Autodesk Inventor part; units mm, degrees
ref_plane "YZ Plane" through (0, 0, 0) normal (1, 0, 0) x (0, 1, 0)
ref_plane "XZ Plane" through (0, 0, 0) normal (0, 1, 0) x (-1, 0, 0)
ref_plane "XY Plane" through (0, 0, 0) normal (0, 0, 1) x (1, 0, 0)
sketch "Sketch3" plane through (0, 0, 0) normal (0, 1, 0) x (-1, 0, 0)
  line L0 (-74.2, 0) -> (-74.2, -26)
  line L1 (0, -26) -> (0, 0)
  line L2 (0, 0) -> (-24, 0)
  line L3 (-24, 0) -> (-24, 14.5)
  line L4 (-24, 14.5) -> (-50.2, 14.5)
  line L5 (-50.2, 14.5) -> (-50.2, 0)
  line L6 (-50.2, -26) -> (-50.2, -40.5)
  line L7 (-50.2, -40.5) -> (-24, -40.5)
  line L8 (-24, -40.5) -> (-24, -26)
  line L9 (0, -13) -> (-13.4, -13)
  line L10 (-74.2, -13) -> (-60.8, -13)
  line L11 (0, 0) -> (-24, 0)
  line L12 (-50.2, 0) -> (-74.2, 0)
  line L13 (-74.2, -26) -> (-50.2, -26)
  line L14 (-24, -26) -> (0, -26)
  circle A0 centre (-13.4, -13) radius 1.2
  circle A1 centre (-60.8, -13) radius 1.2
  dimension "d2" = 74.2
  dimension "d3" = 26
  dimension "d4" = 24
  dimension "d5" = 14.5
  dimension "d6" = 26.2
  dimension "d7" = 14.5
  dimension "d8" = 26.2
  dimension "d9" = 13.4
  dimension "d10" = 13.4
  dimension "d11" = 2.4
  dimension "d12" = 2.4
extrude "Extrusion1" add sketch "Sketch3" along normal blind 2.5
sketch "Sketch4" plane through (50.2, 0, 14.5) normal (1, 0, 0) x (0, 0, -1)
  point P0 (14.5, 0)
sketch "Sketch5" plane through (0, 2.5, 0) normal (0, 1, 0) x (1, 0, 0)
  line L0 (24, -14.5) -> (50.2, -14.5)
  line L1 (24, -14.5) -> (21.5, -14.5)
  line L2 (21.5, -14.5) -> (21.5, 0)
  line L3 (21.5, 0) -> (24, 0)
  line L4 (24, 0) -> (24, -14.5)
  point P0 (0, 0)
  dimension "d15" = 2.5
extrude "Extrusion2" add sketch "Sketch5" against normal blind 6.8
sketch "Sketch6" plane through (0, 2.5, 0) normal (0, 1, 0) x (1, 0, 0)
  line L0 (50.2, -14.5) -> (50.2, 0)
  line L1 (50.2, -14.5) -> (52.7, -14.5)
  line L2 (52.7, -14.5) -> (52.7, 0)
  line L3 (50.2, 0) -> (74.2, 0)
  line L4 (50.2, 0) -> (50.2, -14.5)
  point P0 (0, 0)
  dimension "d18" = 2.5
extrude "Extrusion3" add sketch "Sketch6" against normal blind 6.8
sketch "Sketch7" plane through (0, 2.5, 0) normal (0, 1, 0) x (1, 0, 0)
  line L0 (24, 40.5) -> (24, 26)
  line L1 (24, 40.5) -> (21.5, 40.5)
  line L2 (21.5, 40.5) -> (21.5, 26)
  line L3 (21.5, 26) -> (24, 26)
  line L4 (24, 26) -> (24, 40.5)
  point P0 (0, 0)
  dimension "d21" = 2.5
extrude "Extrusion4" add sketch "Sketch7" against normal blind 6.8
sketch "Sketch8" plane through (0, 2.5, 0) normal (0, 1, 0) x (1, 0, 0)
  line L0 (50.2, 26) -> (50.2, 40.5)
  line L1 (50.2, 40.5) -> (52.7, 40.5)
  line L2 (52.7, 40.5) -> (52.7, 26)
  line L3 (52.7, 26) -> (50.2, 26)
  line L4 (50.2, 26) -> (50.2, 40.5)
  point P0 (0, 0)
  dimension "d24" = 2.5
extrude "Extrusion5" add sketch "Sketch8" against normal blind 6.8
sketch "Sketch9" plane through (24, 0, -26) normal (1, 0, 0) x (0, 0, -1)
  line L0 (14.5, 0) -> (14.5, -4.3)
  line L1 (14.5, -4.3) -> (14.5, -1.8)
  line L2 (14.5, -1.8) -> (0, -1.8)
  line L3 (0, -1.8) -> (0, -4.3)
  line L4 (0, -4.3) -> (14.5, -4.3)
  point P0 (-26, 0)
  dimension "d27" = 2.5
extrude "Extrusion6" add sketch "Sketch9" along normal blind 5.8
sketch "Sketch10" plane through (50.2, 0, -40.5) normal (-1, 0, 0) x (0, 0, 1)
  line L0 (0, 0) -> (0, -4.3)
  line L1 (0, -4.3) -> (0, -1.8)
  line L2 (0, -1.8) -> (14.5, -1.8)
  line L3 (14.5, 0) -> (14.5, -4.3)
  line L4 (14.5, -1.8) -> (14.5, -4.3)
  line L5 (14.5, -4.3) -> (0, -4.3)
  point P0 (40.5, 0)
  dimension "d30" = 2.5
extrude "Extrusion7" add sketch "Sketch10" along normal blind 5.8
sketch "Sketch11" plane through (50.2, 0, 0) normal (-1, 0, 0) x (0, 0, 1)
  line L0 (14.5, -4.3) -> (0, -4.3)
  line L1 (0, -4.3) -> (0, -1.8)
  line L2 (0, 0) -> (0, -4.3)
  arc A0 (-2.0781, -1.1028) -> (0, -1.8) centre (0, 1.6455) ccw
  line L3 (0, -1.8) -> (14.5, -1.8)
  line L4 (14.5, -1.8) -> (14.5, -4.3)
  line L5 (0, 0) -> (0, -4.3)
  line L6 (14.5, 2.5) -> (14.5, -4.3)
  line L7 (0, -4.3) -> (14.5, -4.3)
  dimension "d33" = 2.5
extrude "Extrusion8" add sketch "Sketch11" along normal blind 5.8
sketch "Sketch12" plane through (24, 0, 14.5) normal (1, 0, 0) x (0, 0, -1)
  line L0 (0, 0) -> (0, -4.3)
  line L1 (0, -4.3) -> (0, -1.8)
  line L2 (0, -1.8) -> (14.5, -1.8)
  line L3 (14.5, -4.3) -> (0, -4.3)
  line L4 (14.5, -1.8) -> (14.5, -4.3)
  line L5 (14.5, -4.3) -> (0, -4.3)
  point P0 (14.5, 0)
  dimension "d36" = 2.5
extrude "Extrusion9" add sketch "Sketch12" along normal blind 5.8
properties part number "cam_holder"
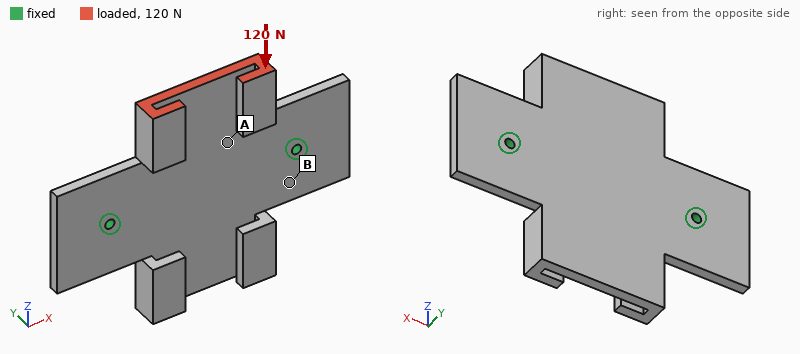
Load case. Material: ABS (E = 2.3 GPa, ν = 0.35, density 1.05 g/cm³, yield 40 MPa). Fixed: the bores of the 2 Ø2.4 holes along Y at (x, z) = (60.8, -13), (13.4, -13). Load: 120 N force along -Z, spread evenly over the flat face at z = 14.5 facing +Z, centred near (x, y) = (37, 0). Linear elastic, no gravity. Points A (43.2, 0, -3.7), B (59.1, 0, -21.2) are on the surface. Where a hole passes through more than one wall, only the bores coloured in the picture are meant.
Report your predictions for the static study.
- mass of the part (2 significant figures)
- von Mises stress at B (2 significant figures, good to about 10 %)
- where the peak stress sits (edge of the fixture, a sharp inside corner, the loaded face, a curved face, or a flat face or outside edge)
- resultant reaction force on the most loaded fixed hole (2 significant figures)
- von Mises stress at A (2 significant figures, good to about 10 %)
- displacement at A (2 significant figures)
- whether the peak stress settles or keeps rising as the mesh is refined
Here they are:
9.0 g
1.9 MPa
edge of the fixture
61 N
3.9 MPa
0.16 mm
keeps rising
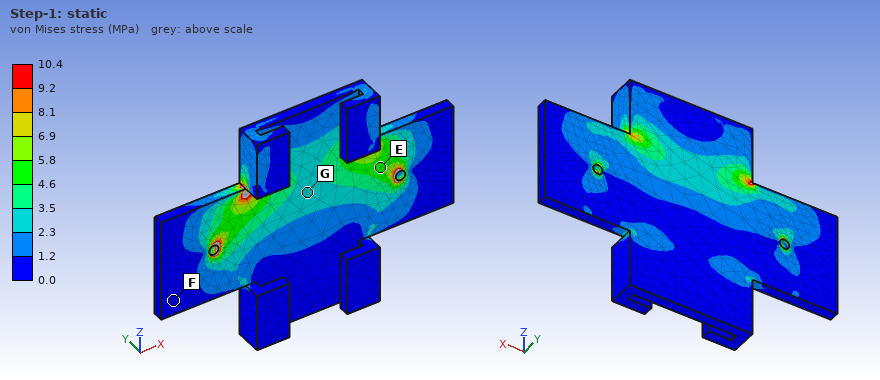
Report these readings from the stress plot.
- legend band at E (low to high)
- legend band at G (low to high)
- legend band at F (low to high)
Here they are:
4.6 to 5.8 MPa
2.3 to 3.5 MPa
0.0 to 1.2 MPa
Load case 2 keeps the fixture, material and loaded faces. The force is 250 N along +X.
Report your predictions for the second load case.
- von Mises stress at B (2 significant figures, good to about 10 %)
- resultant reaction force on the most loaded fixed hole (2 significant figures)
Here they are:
2.2 MPa
190 N
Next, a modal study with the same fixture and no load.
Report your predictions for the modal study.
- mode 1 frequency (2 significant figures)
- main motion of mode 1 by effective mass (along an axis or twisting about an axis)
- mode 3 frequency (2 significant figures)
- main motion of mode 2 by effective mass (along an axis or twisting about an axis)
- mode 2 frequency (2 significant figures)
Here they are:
470 Hz
twisting about X
1300 Hz
along Y
640 Hz
